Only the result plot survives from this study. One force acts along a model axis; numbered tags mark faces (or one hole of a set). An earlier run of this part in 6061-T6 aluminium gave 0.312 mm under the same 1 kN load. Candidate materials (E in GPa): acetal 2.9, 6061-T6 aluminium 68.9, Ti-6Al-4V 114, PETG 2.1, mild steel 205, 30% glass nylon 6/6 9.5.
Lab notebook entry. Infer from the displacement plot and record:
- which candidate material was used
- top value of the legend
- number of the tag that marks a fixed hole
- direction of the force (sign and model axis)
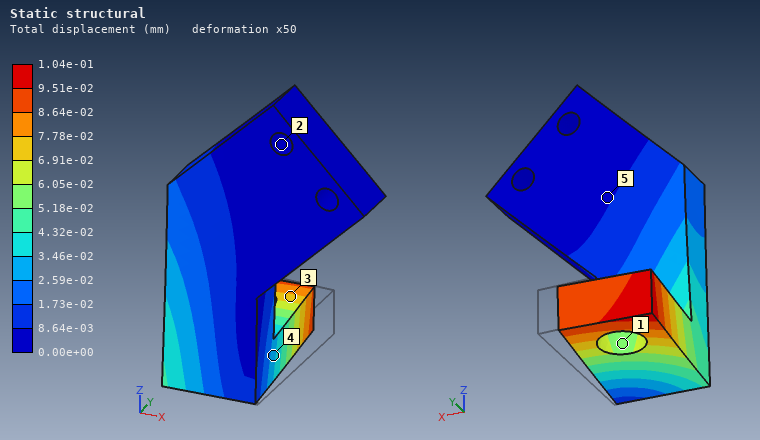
mild steel
1.04e-01 mm
2
-X
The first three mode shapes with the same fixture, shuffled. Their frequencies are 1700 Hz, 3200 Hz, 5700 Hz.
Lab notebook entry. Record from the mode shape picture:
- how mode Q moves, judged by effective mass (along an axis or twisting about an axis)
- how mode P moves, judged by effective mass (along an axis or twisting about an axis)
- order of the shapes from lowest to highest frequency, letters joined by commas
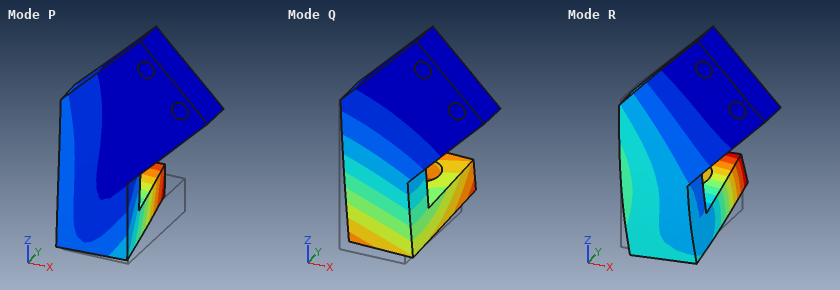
along Y
along X
Q, P, R
